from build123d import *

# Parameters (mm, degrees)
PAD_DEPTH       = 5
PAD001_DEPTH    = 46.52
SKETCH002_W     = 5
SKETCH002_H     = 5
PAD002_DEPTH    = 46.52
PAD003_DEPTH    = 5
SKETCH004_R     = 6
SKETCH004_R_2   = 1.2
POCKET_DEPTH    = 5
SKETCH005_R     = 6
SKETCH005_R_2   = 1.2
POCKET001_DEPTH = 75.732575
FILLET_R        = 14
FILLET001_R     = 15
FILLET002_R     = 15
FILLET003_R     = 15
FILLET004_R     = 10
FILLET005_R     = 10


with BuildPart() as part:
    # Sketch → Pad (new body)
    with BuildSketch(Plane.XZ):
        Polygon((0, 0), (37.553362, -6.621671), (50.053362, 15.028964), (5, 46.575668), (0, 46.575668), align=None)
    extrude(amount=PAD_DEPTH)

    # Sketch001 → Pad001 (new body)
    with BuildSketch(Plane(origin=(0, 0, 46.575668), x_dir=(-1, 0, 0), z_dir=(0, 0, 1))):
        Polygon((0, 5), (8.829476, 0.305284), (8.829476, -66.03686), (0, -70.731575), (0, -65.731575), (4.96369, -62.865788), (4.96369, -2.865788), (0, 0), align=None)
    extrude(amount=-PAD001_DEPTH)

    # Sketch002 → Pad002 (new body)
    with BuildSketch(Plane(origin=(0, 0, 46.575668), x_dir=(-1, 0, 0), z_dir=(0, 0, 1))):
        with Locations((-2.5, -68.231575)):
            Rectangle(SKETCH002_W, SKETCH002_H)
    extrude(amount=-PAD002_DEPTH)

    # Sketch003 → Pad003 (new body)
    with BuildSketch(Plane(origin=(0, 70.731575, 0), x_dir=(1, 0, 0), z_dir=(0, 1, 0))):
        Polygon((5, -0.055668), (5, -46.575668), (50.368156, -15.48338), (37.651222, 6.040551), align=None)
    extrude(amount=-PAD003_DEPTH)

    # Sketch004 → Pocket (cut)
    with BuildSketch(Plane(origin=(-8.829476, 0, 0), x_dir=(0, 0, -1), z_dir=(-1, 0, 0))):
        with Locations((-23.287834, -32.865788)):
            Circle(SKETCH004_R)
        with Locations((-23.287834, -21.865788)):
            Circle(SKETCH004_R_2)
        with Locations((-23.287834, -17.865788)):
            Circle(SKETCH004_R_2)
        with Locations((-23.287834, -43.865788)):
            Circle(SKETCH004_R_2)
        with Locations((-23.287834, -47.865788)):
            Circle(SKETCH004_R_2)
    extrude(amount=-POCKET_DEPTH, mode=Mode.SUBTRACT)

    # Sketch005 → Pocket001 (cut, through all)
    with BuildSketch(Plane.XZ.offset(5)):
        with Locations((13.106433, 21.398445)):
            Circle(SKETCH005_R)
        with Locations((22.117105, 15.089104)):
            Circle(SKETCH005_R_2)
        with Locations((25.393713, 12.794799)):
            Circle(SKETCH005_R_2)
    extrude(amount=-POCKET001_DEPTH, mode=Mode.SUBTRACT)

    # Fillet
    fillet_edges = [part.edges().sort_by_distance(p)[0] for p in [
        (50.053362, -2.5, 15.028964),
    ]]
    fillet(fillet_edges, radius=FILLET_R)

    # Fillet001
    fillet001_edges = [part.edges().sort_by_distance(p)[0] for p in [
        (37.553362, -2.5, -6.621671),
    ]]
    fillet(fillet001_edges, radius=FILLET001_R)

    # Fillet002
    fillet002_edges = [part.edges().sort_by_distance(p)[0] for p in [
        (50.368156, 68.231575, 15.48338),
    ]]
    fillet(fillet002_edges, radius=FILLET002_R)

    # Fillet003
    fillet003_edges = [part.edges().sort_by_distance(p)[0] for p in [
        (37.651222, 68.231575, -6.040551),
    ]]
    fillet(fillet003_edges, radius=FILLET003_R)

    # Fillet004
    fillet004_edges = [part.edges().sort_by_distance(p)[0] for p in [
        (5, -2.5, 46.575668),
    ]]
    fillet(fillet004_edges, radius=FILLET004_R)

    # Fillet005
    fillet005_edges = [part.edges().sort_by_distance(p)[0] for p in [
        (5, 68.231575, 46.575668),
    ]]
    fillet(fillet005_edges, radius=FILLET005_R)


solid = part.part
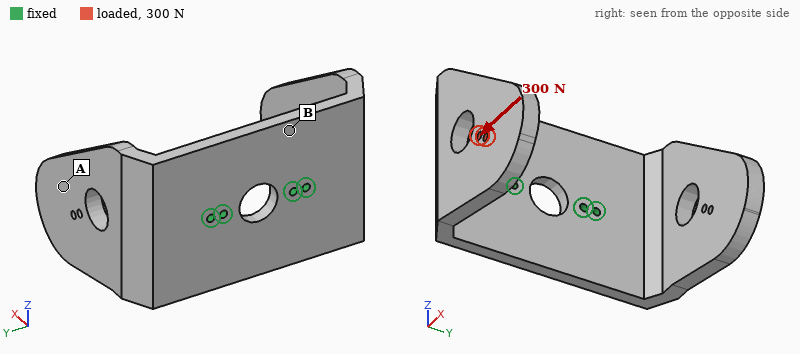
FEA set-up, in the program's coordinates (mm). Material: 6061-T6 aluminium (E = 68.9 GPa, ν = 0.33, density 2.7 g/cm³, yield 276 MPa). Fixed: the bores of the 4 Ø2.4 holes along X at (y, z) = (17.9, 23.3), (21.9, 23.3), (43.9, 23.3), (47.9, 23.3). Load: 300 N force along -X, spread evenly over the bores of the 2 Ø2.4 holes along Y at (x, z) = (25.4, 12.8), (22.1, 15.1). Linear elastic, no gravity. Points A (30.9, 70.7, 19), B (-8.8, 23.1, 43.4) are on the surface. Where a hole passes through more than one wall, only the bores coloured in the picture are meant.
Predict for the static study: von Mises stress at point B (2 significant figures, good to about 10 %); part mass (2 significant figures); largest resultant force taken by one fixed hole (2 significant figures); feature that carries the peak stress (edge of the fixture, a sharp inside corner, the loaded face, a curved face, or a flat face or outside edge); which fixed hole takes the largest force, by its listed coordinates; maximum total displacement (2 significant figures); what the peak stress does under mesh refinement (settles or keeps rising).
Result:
16 MPa
79 g
620 N
edge of the fixture
(17.9, 23.3)
0.34 mm
keeps rising
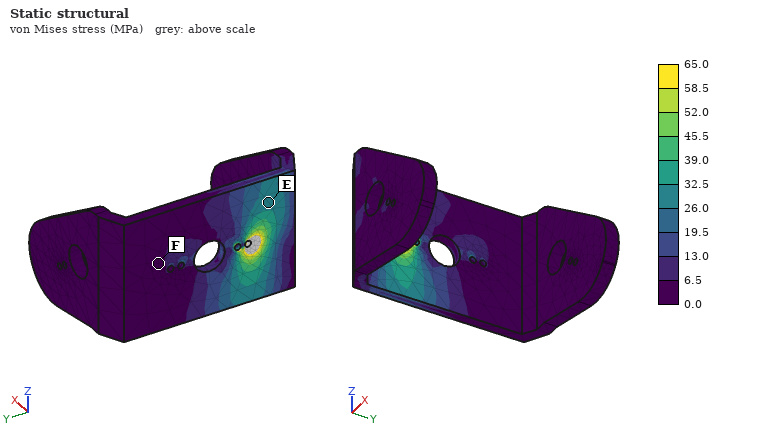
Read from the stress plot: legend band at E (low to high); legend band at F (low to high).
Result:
26.0 to 32.5 MPa
0.0 to 6.5 MPa
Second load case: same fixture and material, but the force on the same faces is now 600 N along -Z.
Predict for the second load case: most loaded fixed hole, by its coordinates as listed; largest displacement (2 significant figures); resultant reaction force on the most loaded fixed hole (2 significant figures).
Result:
(17.9, 23.3)
0.87 mm
790 N
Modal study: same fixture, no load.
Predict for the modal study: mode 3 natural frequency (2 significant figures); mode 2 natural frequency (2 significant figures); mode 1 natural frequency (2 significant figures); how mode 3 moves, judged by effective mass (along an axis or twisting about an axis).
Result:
1100 Hz
860 Hz
830 Hz
along Z
